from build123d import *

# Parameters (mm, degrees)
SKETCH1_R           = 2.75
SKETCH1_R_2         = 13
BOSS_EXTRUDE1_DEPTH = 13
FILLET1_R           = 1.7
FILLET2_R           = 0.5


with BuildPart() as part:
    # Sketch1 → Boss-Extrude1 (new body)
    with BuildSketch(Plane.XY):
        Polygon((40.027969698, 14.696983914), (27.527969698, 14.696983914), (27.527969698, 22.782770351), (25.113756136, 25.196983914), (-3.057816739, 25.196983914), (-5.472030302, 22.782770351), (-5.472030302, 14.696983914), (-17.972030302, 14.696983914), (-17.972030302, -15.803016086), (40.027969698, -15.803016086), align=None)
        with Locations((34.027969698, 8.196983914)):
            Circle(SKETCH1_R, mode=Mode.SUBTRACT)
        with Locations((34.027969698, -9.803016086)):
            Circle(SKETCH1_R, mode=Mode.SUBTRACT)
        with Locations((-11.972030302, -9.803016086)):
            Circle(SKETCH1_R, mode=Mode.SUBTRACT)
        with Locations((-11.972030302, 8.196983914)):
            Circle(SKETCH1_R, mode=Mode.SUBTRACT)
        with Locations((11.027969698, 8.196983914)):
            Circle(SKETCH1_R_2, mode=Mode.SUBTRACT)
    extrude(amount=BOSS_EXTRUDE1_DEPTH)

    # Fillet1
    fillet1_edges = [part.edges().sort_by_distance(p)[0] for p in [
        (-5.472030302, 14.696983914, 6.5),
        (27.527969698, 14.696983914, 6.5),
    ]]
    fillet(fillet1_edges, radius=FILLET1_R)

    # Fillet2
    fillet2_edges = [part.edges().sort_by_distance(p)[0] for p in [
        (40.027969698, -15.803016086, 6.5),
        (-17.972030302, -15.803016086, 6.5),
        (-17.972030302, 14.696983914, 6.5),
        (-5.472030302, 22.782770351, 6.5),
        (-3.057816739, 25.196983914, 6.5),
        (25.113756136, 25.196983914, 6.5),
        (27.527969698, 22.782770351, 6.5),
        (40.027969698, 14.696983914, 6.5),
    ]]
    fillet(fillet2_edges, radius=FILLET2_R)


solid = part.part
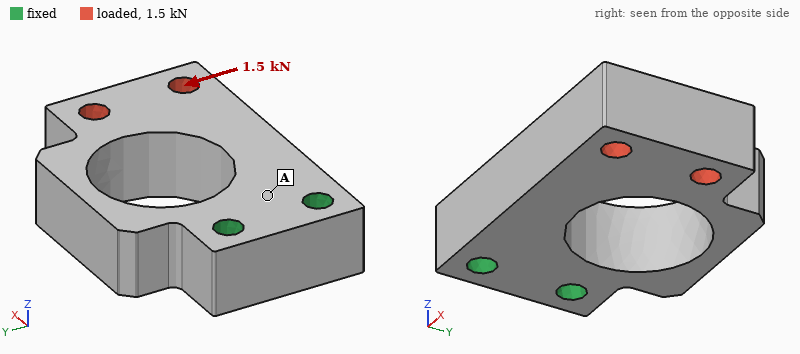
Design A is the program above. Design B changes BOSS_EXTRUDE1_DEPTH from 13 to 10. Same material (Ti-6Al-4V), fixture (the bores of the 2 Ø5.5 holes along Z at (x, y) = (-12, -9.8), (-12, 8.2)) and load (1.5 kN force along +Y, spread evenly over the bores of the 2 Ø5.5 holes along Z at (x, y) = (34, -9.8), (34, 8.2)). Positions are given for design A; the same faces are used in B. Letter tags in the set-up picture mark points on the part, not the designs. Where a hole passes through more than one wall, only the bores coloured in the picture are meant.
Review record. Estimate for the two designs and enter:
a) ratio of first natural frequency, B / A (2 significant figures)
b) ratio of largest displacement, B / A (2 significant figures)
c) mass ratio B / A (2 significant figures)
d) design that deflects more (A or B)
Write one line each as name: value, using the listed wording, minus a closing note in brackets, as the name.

ratio of first natural frequency, B / A: 0.80
ratio of largest displacement, B / A: 1.3
mass ratio B / A: 0.77
design that deflects more: B
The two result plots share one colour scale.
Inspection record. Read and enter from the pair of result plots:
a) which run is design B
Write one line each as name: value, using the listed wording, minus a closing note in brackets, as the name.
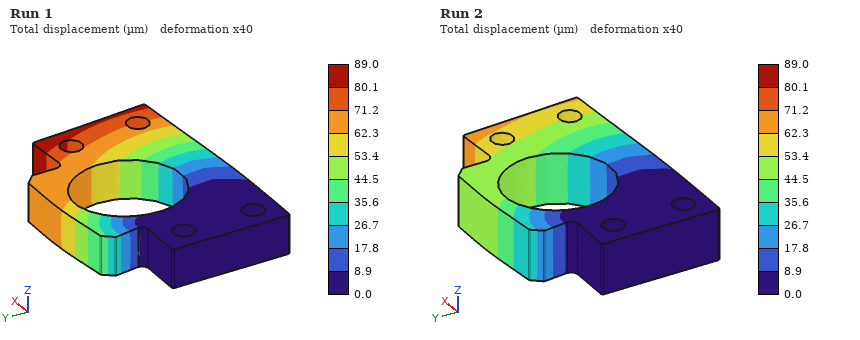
which run is design B: Run 1
